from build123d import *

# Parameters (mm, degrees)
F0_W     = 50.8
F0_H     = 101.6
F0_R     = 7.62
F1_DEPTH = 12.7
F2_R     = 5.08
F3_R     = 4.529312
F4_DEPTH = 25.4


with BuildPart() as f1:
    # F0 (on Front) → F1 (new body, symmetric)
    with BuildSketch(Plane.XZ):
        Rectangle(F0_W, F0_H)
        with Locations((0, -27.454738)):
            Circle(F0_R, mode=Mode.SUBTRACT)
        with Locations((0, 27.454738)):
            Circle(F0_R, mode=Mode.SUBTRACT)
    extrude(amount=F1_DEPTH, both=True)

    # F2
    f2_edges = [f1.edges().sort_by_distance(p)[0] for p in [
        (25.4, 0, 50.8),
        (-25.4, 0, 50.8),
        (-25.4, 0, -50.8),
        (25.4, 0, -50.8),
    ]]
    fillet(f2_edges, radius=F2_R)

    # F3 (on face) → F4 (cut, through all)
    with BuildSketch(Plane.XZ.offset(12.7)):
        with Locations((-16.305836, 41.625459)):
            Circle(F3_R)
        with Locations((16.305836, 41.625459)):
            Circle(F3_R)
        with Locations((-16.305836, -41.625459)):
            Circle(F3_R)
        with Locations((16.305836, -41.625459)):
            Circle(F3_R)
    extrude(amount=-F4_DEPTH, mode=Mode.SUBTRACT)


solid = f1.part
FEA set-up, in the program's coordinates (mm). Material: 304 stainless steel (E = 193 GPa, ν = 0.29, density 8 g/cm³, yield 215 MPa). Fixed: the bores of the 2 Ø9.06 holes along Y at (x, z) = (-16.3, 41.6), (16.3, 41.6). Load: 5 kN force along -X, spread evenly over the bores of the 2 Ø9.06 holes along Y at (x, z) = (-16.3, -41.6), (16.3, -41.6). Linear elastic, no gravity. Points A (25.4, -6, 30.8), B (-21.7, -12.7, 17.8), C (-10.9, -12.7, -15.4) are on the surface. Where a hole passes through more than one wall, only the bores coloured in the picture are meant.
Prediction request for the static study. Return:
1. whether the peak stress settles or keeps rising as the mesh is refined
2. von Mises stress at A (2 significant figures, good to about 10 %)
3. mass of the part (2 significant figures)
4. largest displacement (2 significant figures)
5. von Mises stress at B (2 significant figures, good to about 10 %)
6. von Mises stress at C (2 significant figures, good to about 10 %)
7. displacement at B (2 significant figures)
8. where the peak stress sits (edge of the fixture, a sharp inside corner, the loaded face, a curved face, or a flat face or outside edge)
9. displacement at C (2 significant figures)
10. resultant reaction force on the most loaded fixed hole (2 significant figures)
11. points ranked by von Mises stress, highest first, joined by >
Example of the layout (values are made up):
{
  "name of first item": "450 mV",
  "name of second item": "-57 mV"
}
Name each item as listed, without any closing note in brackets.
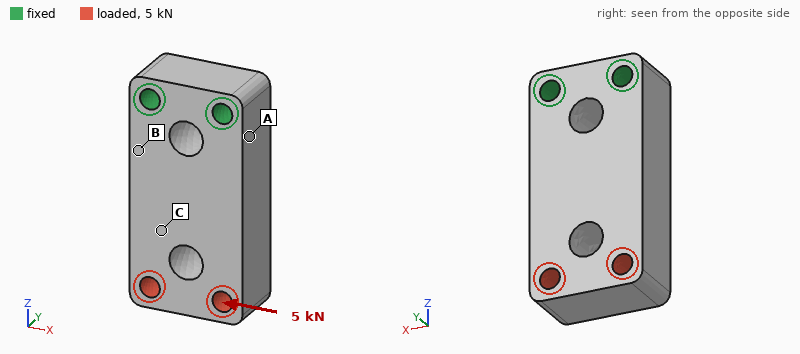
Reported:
{
  "whether the peak stress settles or keeps rising as the mesh is refined": "keeps rising",
  "von Mises stress at A": "31 MPa",
  "mass of the part": "920 g",
  "largest displacement": "29 µm",
  "von Mises stress at B": "21 MPa",
  "von Mises stress at C": "5.9 MPa",
  "displacement at B": "5.6 µm",
  "where the peak stress sits": "edge of the fixture",
  "displacement at C": "14 µm",
  "resultant reaction force on the most loaded fixed hole": "11 kN",
  "points ranked by von Mises stress, highest first, joined by >": "A > B > C"
}
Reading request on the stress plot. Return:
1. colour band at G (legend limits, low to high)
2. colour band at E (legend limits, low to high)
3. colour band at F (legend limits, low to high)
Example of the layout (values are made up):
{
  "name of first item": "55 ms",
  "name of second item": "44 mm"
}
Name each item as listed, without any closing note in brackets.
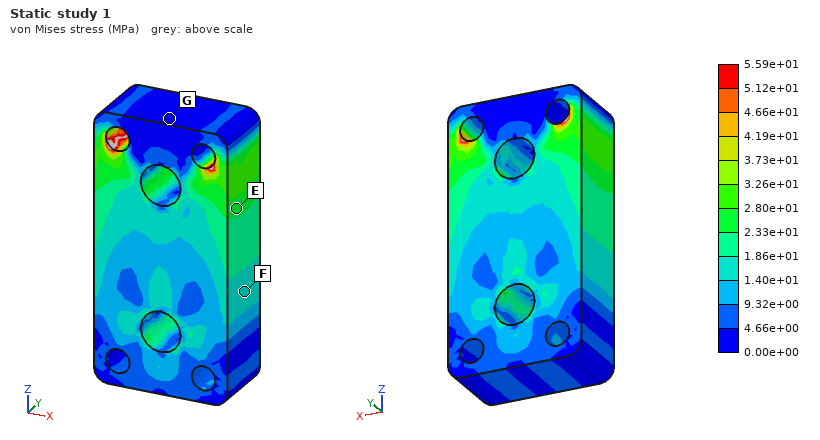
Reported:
{
  "colour band at G": "0.00e+00 to 4.66e+00 MPa",
  "colour band at E": "2.33e+01 to 2.80e+01 MPa",
  "colour band at F": "1.40e+01 to 1.86e+01 MPa"
}
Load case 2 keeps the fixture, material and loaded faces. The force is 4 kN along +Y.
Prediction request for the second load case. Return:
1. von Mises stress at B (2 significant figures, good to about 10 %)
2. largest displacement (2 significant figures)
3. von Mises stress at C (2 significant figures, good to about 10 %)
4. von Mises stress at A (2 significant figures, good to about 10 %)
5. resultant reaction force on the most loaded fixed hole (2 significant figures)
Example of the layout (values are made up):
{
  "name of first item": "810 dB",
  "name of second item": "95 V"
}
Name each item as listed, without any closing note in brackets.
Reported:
{
  "von Mises stress at B": "53 MPa",
  "largest displacement": "84 µm",
  "von Mises stress at C": "23 MPa",
  "von Mises stress at A": "24 MPa",
  "resultant reaction force on the most loaded fixed hole": "2.0 kN"
}
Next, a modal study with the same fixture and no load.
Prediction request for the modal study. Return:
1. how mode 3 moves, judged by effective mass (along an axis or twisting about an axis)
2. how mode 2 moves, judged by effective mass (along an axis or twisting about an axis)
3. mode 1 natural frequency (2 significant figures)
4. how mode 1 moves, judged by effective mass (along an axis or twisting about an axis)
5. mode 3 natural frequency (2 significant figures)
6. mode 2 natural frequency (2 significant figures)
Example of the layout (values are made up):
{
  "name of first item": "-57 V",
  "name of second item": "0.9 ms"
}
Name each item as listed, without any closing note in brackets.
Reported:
{
  "how mode 3 moves, judged by effective mass": "twisting about Z",
  "how mode 2 moves, judged by effective mass": "along X",
  "mode 1 natural frequency": "2300 Hz",
  "how mode 1 moves, judged by effective mass": "along Y",
  "mode 3 natural frequency": "6500 Hz",
  "mode 2 natural frequency": "4100 Hz"
}
